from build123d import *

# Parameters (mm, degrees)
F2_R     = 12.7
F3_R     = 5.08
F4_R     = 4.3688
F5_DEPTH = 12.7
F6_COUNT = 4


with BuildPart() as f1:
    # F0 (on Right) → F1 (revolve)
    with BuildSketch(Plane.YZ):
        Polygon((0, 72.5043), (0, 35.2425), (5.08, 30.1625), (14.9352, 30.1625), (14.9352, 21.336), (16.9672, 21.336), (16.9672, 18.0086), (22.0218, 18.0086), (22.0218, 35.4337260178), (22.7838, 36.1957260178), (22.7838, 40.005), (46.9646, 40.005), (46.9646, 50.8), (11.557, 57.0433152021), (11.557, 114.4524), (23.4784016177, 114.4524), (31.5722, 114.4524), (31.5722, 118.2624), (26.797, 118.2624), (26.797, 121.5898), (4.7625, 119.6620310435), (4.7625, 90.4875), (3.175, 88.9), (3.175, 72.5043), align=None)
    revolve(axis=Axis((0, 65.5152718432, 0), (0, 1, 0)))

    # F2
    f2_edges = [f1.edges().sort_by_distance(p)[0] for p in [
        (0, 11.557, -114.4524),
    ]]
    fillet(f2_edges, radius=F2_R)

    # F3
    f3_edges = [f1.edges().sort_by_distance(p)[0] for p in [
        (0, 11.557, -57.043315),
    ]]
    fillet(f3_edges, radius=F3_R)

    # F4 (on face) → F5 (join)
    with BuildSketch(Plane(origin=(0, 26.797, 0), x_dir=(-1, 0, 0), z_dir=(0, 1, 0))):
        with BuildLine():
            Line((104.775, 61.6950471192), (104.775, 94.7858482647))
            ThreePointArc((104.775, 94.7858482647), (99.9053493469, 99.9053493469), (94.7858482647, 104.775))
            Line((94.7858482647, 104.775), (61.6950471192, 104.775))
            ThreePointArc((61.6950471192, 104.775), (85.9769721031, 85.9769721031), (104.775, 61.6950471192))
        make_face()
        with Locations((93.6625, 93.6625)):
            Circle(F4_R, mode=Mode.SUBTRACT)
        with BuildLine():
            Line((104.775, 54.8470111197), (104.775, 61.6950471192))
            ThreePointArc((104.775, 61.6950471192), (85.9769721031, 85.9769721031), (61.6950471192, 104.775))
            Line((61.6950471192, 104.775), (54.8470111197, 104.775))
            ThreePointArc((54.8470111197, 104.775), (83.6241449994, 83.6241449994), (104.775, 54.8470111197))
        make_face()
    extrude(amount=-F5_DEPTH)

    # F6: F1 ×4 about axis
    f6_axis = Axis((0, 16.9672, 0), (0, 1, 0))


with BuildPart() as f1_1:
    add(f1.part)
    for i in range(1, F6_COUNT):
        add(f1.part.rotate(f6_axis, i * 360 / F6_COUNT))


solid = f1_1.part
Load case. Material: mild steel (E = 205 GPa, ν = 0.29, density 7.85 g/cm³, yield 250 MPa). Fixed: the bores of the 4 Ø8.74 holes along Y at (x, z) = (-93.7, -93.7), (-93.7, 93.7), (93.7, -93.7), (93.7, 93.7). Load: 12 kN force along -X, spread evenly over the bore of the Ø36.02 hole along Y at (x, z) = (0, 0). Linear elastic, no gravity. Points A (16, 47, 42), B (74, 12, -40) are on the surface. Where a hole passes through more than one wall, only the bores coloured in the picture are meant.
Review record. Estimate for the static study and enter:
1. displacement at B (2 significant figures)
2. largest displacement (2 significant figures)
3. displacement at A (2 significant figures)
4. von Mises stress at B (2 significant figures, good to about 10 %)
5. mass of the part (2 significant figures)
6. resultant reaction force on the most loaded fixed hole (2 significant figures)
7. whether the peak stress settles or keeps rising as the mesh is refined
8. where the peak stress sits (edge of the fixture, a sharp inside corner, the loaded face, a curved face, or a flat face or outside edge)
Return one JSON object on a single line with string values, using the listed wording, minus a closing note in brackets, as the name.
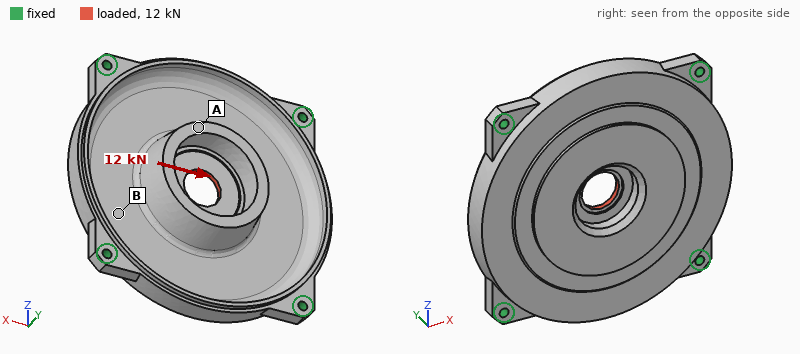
{"displacement at B": "12 µm", "largest displacement": "19 µm", "displacement at A": "16 µm", "von Mises stress at B": "10 MPa", "mass of the part": "5.4 kg", "resultant reaction force on the most loaded fixed hole": "3.0 kN", "whether the peak stress settles or keeps rising as the mesh is refined": "keeps rising", "where the peak stress sits": "edge of the fixture"}
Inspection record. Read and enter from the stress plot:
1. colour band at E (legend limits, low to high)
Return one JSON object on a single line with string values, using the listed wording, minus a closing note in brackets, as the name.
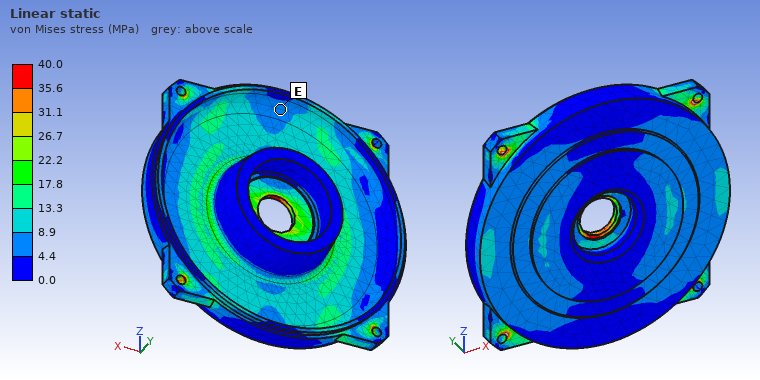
{"colour band at E": "4.4 to 8.9 MPa"}
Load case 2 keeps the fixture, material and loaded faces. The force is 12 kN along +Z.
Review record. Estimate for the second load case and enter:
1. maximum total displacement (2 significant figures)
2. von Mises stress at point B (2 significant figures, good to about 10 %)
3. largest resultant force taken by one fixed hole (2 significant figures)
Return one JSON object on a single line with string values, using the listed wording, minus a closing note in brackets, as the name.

{"maximum total displacement": "19 µm", "von Mises stress at point B": "12 MPa", "largest resultant force taken by one fixed hole": "3.0 kN"}
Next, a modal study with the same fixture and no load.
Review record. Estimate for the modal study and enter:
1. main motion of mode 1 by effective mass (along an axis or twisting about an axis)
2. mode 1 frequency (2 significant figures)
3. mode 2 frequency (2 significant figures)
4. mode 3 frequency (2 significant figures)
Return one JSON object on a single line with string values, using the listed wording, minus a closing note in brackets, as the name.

{"main motion of mode 1 by effective mass": "along Y", "mode 1 frequency": "1300 Hz", "mode 2 frequency": "2000 Hz", "mode 3 frequency": "2000 Hz"}
